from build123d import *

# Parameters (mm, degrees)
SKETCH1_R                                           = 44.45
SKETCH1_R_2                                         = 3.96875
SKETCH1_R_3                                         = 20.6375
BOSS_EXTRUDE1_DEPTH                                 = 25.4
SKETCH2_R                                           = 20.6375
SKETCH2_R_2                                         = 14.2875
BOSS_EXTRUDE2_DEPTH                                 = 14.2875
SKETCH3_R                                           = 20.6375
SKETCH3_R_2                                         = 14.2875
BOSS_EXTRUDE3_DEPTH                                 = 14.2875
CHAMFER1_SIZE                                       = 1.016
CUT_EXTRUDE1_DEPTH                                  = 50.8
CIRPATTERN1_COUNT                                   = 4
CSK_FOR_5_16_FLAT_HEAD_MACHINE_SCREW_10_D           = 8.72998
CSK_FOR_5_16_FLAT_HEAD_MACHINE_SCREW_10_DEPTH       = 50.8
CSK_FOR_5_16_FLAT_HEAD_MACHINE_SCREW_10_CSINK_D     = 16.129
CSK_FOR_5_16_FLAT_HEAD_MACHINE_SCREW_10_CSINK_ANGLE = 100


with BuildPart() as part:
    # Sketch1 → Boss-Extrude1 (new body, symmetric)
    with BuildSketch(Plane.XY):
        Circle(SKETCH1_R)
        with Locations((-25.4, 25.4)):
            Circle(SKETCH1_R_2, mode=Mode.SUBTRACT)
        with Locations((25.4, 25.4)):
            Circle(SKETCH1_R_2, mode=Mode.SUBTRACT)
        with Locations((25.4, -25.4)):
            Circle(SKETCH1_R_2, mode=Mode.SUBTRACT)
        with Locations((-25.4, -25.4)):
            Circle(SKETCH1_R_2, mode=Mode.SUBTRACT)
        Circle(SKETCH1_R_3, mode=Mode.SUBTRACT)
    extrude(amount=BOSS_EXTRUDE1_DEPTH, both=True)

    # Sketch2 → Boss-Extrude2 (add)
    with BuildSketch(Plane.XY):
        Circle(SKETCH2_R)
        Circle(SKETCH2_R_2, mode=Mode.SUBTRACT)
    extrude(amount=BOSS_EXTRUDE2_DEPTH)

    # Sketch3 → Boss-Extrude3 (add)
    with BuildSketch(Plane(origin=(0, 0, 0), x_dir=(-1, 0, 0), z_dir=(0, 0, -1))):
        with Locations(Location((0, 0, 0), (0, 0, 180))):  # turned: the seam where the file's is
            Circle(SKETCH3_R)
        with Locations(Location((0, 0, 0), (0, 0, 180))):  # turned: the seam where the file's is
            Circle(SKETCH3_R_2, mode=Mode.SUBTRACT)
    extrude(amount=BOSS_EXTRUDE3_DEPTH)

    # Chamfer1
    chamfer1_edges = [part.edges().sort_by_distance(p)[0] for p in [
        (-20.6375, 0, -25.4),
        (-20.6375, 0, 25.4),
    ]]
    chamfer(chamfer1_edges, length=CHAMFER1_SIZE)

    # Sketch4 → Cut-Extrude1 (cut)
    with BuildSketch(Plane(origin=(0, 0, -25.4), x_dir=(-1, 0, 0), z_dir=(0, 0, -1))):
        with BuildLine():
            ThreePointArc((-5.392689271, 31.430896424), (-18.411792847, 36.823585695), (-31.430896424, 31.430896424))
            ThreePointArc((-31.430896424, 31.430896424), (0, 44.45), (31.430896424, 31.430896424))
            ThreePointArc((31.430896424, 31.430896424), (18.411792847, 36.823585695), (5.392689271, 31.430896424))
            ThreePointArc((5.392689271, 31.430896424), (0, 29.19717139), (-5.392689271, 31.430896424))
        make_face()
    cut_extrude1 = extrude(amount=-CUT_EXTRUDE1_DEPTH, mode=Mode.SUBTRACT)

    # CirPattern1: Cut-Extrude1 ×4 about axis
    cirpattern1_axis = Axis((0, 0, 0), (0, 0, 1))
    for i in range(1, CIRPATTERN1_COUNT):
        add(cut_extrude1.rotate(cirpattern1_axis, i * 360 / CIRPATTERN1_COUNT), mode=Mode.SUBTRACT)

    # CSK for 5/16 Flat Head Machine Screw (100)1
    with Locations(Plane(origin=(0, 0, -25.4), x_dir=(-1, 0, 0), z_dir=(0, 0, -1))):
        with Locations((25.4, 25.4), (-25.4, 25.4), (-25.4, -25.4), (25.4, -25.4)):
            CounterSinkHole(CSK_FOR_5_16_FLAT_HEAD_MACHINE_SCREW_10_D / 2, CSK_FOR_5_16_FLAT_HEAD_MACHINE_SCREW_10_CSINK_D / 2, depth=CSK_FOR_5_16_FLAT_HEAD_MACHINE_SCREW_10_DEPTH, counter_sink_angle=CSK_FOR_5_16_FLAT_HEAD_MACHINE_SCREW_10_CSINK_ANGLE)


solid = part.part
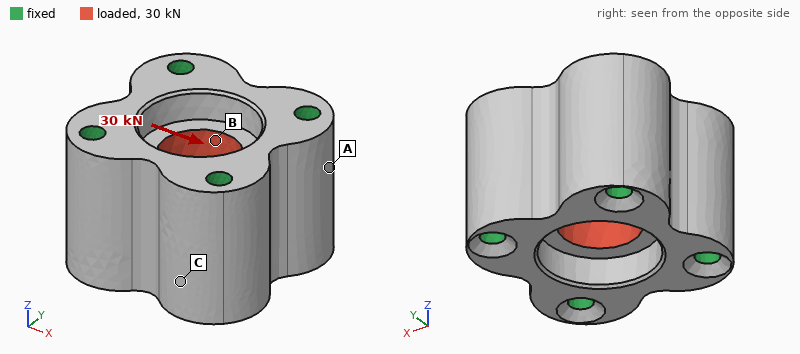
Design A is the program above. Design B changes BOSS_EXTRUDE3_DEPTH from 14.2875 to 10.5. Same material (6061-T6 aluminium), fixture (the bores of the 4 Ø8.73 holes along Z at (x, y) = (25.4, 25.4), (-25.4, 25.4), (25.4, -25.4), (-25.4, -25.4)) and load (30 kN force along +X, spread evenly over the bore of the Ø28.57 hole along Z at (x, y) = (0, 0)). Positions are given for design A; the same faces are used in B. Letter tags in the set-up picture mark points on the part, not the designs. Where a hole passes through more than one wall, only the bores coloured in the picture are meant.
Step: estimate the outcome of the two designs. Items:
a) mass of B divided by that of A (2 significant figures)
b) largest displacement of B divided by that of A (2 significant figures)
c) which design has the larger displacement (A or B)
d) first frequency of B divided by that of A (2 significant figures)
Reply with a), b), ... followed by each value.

a) 0.98
b) 1.1
c) B
d) 0.99
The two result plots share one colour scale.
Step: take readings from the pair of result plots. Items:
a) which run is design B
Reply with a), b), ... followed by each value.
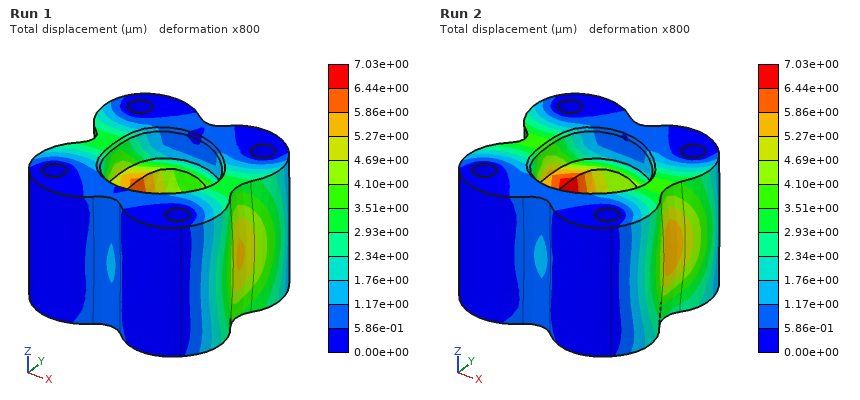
a) Run 2
